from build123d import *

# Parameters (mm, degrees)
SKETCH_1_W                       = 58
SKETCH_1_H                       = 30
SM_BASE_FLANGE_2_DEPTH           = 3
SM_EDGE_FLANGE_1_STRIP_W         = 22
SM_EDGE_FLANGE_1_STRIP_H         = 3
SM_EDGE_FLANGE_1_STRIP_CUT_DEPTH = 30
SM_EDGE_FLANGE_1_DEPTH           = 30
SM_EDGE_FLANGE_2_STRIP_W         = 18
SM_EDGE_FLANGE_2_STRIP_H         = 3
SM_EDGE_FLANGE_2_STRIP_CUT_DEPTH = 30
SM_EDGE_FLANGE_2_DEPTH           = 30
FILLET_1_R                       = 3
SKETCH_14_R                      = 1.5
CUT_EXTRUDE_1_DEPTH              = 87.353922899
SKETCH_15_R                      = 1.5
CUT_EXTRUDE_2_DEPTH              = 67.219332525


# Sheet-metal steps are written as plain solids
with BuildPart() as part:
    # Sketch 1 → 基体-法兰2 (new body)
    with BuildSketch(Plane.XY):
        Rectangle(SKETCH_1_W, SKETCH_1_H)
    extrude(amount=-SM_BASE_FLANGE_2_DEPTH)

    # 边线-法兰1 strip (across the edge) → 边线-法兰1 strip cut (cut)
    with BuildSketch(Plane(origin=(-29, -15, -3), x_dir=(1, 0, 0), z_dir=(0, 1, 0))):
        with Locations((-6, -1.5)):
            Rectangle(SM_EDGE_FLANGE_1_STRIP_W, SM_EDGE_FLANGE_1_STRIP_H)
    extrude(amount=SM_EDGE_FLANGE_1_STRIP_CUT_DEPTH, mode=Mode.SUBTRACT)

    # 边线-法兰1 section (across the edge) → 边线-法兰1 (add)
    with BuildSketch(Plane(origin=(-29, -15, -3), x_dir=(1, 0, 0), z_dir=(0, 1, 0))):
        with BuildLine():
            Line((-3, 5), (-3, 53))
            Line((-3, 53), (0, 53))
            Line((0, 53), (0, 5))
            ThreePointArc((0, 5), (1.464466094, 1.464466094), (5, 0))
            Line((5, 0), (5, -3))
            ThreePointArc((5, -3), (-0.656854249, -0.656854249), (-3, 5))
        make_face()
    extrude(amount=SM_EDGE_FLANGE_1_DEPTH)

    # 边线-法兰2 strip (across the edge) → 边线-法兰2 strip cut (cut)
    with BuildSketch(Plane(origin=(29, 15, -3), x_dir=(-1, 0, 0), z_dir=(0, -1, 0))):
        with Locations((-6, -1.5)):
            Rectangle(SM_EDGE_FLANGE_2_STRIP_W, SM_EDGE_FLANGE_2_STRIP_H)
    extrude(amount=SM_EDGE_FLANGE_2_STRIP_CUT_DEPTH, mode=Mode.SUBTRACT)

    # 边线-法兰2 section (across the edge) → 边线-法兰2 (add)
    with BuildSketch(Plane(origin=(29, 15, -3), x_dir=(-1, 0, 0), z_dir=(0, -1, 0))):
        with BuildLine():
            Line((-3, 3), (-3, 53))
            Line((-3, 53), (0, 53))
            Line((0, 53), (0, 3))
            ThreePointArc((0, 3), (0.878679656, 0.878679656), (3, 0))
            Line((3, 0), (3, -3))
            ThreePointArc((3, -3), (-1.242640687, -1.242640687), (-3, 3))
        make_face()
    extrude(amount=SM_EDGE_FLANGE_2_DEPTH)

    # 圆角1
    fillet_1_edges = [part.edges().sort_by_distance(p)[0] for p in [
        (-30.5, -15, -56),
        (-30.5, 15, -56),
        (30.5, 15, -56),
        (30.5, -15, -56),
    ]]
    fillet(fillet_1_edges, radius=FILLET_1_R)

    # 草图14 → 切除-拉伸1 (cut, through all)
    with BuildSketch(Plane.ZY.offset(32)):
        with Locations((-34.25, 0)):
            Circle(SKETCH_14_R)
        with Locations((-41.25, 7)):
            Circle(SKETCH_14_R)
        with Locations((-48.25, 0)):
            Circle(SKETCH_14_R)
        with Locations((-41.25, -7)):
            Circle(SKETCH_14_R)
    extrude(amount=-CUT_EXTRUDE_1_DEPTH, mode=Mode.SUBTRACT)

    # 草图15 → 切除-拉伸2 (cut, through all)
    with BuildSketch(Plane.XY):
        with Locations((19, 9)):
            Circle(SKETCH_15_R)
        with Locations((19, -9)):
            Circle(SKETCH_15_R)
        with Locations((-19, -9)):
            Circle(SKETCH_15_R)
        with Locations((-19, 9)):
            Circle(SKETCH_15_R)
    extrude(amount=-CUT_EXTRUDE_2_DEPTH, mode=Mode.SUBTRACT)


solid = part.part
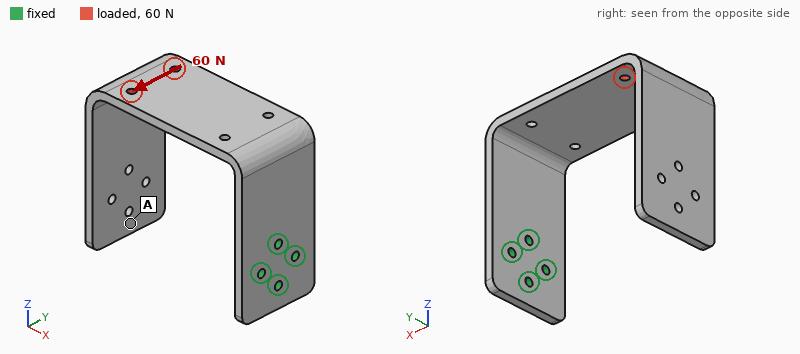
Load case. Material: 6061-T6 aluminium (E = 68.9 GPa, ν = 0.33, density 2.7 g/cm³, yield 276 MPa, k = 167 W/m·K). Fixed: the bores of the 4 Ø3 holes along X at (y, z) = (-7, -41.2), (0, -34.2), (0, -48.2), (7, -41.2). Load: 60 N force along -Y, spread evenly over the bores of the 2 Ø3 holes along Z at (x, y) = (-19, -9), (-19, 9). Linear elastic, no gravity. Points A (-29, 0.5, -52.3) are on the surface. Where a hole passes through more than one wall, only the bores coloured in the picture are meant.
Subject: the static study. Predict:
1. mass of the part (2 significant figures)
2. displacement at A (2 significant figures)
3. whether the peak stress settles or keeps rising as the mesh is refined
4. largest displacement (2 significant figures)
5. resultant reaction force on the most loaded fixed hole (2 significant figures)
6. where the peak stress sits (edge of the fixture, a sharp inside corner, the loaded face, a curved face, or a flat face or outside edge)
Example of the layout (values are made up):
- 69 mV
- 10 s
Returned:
- 39 g
- 0.87 mm
- keeps rising
- 0.93 mm
- 120 N
- edge of the fixture
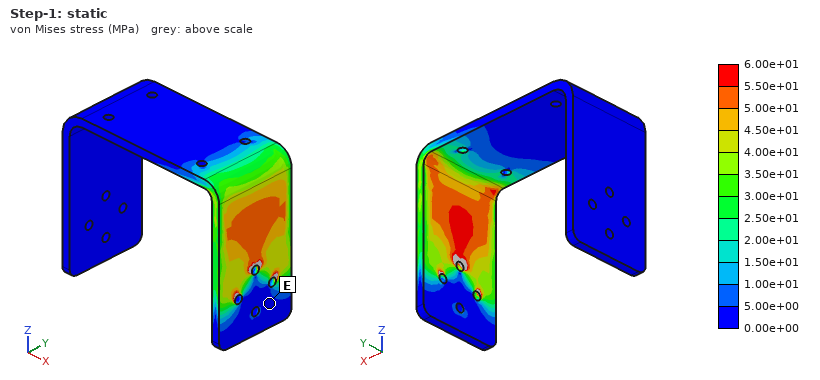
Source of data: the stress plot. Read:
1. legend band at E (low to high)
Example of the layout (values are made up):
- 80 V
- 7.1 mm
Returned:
- 0.00e+00 to 5.00e+00 MPa
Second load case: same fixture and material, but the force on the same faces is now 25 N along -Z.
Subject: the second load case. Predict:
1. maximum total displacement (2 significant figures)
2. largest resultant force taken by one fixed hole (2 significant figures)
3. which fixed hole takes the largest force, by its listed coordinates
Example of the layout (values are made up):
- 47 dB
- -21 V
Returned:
- 1.0 mm
- 95 N
- (0, -34.2)
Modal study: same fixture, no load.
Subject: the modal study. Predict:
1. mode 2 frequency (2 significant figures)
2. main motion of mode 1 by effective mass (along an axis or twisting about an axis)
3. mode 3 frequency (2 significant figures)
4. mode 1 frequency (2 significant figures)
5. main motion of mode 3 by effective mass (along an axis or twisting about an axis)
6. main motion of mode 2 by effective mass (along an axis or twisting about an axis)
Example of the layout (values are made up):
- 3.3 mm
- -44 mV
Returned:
- 260 Hz
- along Z
- 480 Hz
- 180 Hz
- along X
- along Y
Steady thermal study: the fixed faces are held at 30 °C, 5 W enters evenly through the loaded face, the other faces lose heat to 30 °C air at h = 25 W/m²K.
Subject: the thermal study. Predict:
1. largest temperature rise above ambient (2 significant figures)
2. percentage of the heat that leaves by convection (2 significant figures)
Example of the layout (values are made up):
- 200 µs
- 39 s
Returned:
- 16 K
- 50 %
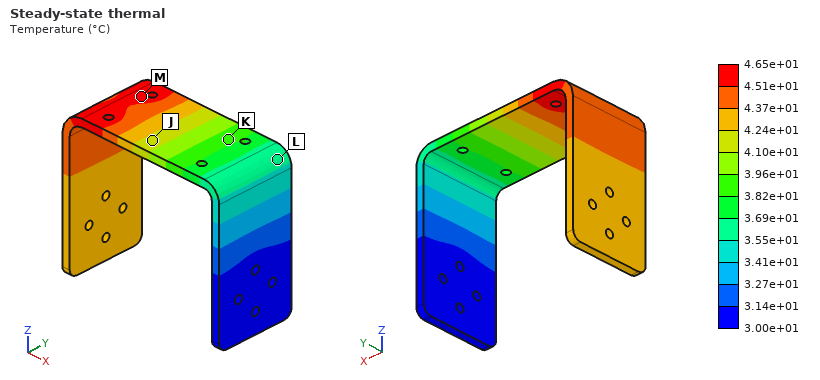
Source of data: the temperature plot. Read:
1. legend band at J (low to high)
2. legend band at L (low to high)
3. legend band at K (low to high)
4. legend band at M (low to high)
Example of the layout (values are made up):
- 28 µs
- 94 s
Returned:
- 4.10e+01 to 4.24e+01 °C
- 3.55e+01 to 3.69e+01 °C
- 3.82e+01 to 3.96e+01 °C
- 4.51e+01 to 4.65e+01 °C
